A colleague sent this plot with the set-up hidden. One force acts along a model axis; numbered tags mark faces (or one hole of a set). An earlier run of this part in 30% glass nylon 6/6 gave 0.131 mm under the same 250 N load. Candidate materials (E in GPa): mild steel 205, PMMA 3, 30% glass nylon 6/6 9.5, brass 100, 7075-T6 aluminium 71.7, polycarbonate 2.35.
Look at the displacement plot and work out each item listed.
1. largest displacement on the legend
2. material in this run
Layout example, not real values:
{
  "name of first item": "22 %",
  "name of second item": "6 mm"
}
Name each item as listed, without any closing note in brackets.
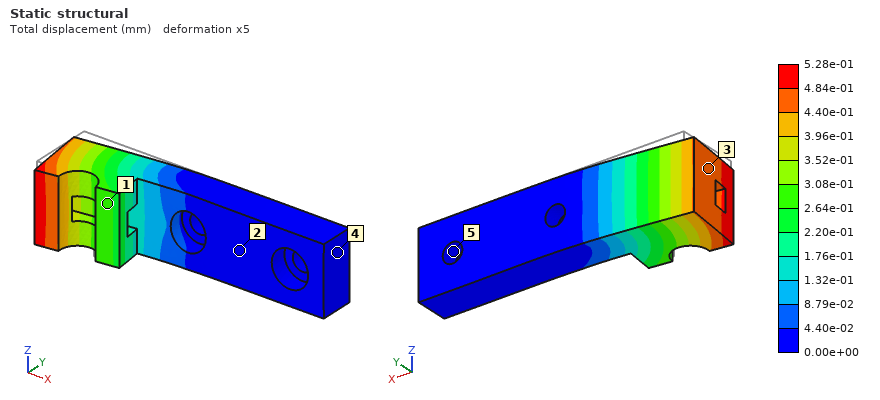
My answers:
{
  "largest displacement on the legend": "5.28e-01 mm",
  "material in this run": "polycarbonate"
}
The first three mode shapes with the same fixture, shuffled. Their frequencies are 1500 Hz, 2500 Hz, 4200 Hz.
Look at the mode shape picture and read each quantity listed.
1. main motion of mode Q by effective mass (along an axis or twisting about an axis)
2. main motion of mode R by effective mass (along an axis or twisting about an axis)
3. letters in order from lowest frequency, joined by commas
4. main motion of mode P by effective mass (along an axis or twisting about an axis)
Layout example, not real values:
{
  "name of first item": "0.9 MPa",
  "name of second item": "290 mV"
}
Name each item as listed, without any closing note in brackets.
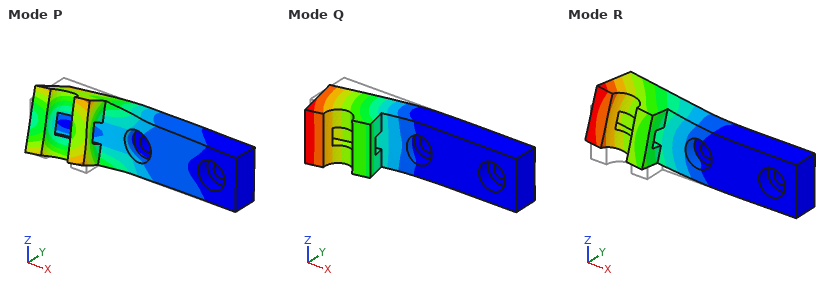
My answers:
{
  "main motion of mode Q by effective mass": "along Y",
  "main motion of mode R by effective mass": "along Z",
  "letters in order from lowest frequency, joined by commas": "Q, R, P",
  "main motion of mode P by effective mass": "twisting about X"
}
